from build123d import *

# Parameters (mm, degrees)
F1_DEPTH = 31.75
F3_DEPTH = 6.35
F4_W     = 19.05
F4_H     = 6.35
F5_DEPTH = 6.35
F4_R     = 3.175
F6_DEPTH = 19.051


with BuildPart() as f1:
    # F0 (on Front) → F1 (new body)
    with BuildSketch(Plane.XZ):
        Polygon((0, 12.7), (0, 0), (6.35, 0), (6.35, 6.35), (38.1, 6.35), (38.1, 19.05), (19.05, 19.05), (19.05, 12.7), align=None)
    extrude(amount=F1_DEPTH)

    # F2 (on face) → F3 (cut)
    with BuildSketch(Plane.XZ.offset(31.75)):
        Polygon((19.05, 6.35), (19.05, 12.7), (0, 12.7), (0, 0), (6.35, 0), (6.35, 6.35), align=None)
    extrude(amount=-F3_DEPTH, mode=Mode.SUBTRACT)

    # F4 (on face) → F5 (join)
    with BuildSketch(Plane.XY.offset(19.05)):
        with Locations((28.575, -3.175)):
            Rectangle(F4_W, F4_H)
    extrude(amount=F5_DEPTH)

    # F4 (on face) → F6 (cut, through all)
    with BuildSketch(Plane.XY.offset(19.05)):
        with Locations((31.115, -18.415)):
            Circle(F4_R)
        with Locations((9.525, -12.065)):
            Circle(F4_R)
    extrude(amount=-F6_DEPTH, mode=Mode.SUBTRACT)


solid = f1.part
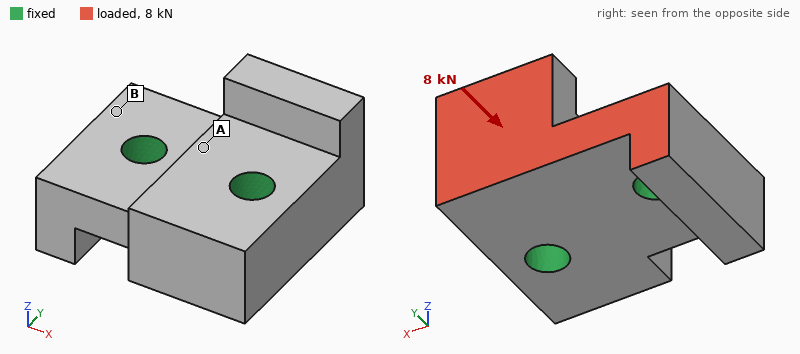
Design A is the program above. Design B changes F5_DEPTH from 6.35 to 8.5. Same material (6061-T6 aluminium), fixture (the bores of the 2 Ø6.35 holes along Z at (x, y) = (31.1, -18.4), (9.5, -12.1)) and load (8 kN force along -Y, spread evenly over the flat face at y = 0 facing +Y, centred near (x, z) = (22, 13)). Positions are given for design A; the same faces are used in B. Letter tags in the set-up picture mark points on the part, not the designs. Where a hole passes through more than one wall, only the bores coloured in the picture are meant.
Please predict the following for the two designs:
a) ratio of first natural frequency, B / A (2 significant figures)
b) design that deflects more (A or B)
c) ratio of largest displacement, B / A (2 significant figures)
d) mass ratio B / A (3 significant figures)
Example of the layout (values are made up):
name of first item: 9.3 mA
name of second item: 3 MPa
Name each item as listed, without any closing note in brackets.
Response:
ratio of first natural frequency, B / A: 0.90
design that deflects more: B
ratio of largest displacement, B / A: 1.6
mass ratio B / A: 1.02
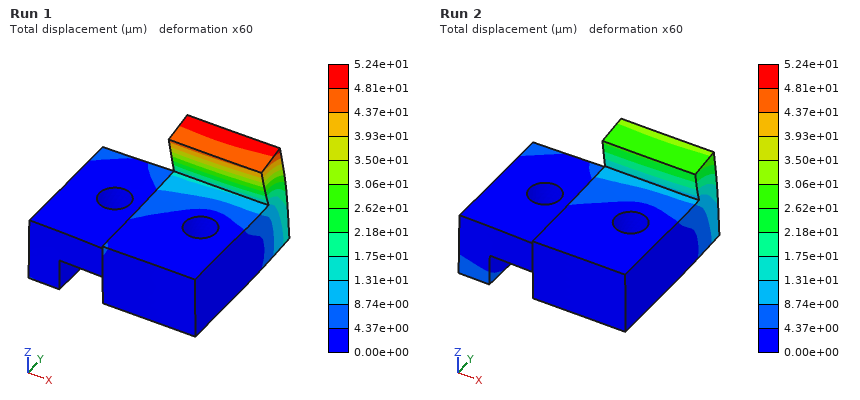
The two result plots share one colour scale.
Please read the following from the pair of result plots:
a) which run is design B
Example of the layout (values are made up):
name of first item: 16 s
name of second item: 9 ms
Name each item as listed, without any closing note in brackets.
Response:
which run is design B: Run 1
